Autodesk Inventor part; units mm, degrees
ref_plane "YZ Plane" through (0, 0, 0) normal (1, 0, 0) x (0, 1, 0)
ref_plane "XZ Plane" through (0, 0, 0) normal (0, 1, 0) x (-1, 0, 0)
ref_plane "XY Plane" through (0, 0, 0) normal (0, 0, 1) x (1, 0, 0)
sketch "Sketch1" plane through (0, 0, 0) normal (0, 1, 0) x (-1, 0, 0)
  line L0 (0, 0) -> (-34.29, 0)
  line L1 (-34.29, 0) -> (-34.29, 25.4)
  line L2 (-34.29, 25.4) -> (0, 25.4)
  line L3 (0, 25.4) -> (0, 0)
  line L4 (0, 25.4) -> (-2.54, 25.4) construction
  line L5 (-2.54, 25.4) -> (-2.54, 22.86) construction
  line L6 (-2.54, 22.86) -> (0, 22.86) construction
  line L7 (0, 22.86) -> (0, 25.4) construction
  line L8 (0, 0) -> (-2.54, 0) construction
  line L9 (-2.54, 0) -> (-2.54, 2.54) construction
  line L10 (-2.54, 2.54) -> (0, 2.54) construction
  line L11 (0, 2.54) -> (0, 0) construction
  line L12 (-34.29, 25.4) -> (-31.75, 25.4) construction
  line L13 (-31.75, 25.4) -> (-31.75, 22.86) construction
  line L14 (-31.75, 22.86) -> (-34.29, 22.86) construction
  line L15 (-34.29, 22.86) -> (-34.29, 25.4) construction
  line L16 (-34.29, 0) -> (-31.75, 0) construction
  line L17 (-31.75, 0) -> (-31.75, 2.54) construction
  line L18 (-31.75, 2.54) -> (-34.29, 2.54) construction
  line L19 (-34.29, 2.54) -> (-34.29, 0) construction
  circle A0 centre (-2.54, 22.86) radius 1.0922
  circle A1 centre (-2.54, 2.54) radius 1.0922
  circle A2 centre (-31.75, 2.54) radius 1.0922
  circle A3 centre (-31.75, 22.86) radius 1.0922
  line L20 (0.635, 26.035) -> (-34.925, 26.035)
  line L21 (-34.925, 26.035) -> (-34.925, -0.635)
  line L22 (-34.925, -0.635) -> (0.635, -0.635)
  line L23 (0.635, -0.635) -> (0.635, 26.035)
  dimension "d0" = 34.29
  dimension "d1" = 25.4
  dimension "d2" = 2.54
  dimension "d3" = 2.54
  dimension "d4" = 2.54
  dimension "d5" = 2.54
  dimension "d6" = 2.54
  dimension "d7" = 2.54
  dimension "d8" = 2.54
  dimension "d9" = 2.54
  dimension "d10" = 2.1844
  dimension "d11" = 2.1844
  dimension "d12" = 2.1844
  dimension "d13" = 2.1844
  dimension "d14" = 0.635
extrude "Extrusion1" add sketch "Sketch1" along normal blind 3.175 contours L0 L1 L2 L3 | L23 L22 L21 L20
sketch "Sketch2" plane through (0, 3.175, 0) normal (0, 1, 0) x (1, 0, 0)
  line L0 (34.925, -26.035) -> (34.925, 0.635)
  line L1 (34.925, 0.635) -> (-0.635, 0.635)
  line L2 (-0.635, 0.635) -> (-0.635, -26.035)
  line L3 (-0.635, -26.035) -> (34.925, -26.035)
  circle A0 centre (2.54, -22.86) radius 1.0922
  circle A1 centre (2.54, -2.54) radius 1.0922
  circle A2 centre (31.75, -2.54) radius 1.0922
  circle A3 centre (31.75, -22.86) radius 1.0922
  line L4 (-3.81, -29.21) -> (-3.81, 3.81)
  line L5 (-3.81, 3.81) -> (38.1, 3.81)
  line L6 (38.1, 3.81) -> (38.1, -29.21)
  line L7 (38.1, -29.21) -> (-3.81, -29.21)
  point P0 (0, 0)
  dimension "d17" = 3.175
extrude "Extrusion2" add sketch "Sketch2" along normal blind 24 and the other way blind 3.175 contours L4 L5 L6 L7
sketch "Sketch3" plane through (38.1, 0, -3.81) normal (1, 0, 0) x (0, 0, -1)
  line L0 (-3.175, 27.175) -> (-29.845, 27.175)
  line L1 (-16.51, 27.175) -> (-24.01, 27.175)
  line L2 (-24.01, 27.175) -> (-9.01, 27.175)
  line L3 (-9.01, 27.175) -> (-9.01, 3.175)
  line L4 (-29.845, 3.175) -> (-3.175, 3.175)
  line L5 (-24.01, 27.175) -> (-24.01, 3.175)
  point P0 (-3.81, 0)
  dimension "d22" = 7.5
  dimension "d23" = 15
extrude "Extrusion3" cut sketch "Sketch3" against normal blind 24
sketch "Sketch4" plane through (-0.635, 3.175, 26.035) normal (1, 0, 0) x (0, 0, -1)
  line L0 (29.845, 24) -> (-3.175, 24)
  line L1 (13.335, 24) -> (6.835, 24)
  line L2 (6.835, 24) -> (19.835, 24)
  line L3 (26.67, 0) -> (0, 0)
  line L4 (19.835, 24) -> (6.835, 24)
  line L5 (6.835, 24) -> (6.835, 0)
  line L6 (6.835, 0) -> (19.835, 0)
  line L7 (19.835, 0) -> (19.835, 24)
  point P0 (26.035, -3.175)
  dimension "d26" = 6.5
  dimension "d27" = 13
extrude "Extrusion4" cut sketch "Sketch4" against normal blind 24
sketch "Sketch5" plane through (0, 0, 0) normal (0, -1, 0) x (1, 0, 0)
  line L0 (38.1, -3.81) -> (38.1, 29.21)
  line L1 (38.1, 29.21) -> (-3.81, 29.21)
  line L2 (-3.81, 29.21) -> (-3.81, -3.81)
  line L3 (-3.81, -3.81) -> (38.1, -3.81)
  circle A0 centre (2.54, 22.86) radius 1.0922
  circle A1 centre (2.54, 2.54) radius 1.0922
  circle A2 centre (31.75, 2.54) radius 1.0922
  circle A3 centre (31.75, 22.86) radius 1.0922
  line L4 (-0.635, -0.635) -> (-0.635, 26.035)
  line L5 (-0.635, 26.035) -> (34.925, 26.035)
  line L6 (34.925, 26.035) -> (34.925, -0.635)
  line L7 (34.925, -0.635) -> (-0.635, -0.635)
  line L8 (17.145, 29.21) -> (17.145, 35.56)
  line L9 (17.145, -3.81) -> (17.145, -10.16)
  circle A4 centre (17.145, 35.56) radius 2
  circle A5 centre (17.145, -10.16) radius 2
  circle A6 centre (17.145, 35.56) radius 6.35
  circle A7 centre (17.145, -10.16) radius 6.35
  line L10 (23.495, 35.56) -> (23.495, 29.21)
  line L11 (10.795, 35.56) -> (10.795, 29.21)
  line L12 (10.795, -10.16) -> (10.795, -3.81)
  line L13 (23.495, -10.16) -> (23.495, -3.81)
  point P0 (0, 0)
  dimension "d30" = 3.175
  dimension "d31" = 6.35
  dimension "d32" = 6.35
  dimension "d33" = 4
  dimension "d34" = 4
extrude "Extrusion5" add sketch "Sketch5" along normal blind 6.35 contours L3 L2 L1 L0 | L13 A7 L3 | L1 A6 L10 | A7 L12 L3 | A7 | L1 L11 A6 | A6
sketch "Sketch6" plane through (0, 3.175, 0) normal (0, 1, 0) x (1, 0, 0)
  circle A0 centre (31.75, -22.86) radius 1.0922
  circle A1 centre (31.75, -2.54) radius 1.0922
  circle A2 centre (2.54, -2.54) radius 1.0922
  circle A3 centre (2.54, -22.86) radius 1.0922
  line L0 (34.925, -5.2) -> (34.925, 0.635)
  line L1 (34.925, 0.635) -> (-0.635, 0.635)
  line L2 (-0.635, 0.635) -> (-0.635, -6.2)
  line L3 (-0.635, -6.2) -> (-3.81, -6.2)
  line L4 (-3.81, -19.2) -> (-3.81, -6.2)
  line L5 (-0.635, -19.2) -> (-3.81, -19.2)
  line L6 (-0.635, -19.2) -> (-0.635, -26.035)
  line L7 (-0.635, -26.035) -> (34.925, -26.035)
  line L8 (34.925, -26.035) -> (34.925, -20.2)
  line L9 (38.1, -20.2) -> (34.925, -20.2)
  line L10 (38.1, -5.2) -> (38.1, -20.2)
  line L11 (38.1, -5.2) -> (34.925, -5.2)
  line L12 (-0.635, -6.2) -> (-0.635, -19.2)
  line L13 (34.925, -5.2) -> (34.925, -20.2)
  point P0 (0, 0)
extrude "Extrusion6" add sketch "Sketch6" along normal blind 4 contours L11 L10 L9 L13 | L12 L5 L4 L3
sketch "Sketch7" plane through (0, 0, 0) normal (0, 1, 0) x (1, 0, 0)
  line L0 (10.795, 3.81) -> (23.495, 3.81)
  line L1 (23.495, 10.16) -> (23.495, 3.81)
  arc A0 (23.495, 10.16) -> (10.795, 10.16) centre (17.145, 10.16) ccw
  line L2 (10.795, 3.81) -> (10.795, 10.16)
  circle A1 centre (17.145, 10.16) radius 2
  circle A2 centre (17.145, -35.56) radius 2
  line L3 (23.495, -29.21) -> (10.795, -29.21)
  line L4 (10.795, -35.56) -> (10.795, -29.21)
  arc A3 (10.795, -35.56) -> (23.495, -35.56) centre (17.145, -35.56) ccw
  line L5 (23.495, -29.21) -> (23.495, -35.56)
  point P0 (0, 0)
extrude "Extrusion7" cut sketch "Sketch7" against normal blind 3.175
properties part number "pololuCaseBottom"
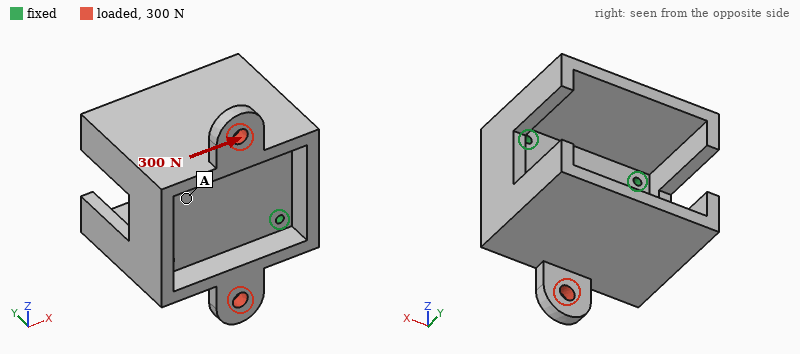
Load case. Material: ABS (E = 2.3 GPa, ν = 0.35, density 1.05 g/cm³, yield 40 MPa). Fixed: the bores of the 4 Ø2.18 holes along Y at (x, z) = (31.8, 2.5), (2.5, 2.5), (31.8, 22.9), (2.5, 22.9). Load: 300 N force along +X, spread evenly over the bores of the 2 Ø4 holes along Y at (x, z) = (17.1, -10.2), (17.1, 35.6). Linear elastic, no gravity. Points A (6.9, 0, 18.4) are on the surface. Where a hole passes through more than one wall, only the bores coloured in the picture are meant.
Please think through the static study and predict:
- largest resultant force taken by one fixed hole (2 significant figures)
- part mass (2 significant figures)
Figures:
89 N
17 g
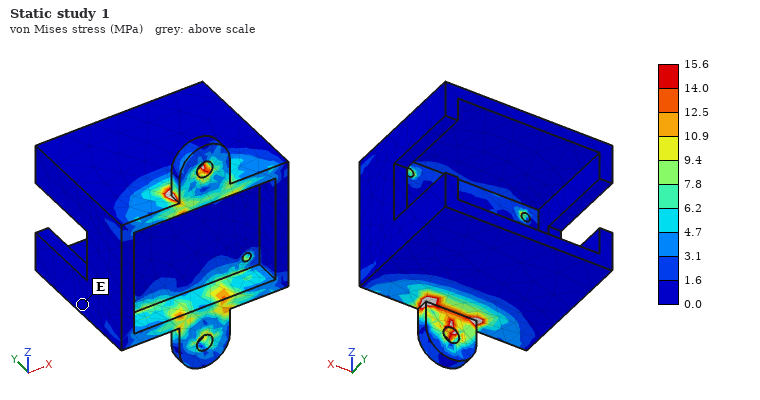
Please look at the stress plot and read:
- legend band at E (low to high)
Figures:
0.0 to 1.6 MPa
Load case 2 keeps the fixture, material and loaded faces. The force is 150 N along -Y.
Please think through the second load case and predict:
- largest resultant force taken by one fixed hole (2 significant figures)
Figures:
38 N
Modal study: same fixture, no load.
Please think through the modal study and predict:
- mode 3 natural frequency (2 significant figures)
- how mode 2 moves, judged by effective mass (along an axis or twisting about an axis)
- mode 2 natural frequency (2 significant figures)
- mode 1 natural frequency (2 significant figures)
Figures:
2500 Hz
along Z
1800 Hz
1700 Hz
